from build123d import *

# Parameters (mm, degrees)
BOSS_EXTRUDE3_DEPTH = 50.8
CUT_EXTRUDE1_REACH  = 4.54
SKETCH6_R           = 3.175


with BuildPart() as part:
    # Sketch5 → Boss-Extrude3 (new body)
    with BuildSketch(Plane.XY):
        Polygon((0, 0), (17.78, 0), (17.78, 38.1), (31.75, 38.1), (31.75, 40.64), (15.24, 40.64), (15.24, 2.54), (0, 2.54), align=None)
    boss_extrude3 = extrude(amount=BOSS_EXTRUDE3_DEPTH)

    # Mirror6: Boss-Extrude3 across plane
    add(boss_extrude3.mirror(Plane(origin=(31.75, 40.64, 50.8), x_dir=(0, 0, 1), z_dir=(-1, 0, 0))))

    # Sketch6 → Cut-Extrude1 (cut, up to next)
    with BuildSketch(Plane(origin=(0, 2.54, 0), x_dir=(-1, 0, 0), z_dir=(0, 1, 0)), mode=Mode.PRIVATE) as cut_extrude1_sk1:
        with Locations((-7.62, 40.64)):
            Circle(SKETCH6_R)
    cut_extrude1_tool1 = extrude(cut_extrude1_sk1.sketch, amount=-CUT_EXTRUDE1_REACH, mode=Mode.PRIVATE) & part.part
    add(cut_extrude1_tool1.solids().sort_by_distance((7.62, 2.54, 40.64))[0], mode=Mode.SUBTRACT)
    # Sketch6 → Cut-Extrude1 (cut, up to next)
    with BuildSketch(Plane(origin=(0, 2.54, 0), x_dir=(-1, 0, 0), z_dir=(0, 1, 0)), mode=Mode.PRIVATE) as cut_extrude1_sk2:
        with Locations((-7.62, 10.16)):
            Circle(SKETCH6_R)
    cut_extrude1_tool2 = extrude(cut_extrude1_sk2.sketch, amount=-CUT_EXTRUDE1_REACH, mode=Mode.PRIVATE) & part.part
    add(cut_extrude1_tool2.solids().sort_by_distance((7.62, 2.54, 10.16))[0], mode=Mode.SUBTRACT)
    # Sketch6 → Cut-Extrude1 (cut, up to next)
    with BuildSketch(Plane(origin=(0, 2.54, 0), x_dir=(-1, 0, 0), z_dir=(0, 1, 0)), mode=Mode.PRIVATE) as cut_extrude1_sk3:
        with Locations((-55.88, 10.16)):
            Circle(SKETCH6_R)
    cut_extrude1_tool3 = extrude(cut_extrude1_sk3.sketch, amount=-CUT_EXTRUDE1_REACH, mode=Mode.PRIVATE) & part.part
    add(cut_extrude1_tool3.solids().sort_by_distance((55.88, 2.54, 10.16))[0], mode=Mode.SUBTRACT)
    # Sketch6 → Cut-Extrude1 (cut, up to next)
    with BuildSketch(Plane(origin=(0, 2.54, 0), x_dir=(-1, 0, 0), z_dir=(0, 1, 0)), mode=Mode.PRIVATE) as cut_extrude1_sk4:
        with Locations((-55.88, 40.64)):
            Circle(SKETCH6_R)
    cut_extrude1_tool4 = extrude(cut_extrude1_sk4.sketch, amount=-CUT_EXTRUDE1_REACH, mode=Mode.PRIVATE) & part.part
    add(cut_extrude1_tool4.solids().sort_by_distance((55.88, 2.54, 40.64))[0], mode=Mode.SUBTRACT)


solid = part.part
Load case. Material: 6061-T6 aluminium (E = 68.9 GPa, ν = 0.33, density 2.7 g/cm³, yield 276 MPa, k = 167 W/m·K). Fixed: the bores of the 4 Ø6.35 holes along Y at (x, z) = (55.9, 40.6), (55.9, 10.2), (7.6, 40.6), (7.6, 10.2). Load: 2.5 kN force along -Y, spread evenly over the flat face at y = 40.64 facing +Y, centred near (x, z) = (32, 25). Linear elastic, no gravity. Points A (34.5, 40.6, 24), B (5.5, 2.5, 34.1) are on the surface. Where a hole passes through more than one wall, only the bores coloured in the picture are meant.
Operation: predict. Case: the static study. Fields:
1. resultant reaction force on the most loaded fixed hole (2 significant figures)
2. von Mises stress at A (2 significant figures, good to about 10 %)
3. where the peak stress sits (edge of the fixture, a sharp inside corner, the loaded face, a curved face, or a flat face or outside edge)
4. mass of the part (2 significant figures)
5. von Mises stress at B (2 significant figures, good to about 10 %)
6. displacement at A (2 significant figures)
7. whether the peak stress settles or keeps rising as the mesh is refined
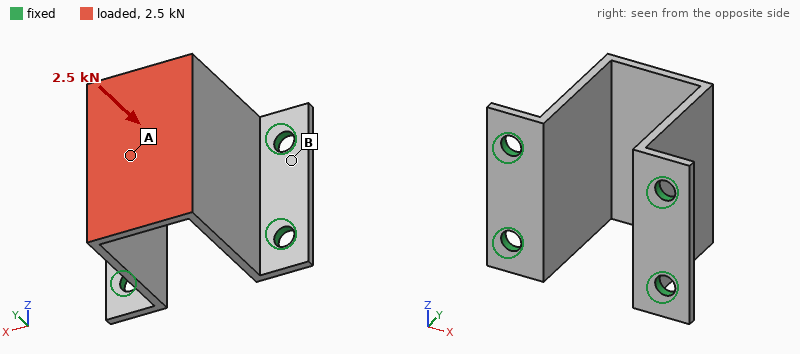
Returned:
630 N
70 MPa
edge of the fixture
48 g
22 MPa
0.096 mm
keeps rising
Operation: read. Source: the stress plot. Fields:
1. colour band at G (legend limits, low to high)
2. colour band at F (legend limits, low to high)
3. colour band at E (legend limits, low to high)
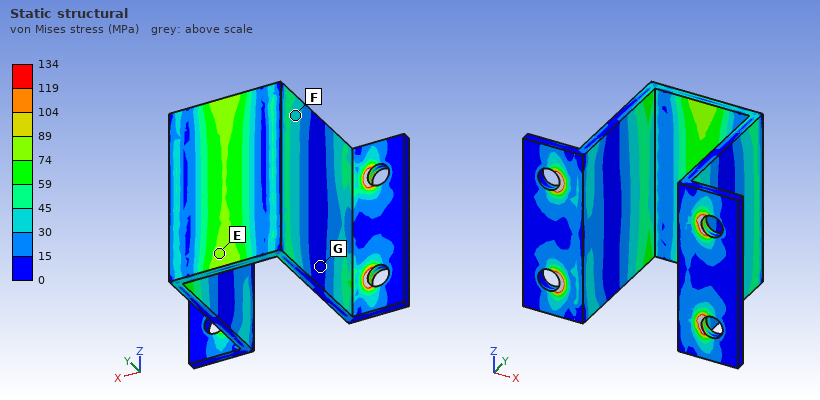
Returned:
0 to 15 MPa
30 to 45 MPa
74 to 89 MPa
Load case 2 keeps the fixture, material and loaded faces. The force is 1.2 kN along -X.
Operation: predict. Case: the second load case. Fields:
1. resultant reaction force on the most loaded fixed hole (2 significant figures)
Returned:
510 N
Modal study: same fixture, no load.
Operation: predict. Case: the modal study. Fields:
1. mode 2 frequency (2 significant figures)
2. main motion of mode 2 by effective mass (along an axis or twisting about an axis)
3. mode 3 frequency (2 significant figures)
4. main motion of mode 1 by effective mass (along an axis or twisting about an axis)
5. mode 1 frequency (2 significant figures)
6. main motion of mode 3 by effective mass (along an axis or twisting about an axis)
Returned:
3000 Hz
twisting about Y
3700 Hz
along X
1300 Hz
along Z
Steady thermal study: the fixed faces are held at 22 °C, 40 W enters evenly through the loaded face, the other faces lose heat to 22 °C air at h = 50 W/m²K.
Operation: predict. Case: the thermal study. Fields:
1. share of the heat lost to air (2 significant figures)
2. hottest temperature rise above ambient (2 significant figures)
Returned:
28 %
39 K
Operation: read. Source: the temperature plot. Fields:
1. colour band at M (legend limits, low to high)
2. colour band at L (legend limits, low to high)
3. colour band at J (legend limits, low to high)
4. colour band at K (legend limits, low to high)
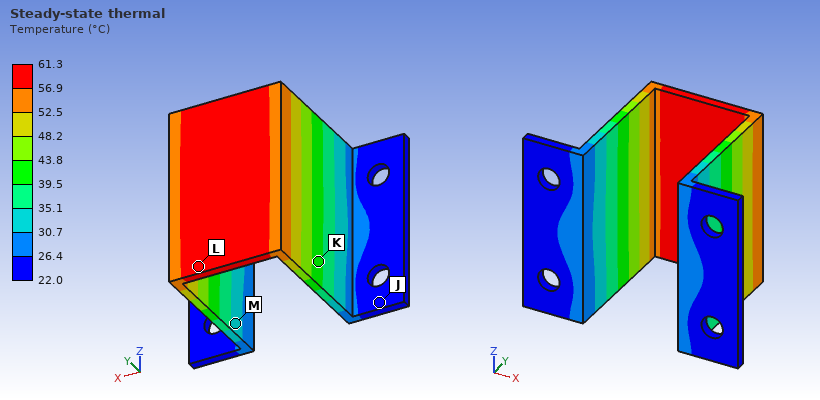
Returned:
30.7 to 35.1 °C
56.9 to 61.3 °C
22.0 to 26.4 °C
39.5 to 43.8 °C
